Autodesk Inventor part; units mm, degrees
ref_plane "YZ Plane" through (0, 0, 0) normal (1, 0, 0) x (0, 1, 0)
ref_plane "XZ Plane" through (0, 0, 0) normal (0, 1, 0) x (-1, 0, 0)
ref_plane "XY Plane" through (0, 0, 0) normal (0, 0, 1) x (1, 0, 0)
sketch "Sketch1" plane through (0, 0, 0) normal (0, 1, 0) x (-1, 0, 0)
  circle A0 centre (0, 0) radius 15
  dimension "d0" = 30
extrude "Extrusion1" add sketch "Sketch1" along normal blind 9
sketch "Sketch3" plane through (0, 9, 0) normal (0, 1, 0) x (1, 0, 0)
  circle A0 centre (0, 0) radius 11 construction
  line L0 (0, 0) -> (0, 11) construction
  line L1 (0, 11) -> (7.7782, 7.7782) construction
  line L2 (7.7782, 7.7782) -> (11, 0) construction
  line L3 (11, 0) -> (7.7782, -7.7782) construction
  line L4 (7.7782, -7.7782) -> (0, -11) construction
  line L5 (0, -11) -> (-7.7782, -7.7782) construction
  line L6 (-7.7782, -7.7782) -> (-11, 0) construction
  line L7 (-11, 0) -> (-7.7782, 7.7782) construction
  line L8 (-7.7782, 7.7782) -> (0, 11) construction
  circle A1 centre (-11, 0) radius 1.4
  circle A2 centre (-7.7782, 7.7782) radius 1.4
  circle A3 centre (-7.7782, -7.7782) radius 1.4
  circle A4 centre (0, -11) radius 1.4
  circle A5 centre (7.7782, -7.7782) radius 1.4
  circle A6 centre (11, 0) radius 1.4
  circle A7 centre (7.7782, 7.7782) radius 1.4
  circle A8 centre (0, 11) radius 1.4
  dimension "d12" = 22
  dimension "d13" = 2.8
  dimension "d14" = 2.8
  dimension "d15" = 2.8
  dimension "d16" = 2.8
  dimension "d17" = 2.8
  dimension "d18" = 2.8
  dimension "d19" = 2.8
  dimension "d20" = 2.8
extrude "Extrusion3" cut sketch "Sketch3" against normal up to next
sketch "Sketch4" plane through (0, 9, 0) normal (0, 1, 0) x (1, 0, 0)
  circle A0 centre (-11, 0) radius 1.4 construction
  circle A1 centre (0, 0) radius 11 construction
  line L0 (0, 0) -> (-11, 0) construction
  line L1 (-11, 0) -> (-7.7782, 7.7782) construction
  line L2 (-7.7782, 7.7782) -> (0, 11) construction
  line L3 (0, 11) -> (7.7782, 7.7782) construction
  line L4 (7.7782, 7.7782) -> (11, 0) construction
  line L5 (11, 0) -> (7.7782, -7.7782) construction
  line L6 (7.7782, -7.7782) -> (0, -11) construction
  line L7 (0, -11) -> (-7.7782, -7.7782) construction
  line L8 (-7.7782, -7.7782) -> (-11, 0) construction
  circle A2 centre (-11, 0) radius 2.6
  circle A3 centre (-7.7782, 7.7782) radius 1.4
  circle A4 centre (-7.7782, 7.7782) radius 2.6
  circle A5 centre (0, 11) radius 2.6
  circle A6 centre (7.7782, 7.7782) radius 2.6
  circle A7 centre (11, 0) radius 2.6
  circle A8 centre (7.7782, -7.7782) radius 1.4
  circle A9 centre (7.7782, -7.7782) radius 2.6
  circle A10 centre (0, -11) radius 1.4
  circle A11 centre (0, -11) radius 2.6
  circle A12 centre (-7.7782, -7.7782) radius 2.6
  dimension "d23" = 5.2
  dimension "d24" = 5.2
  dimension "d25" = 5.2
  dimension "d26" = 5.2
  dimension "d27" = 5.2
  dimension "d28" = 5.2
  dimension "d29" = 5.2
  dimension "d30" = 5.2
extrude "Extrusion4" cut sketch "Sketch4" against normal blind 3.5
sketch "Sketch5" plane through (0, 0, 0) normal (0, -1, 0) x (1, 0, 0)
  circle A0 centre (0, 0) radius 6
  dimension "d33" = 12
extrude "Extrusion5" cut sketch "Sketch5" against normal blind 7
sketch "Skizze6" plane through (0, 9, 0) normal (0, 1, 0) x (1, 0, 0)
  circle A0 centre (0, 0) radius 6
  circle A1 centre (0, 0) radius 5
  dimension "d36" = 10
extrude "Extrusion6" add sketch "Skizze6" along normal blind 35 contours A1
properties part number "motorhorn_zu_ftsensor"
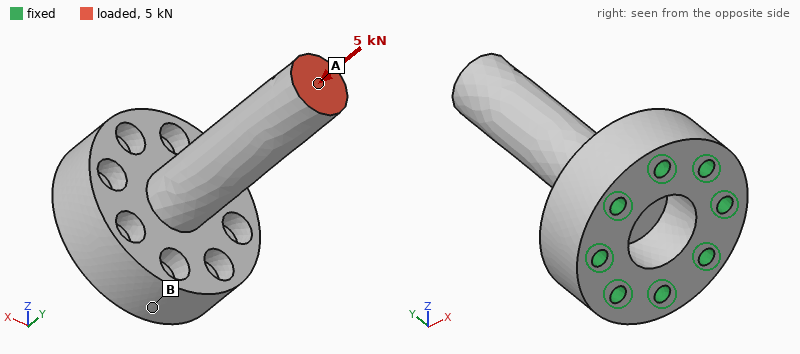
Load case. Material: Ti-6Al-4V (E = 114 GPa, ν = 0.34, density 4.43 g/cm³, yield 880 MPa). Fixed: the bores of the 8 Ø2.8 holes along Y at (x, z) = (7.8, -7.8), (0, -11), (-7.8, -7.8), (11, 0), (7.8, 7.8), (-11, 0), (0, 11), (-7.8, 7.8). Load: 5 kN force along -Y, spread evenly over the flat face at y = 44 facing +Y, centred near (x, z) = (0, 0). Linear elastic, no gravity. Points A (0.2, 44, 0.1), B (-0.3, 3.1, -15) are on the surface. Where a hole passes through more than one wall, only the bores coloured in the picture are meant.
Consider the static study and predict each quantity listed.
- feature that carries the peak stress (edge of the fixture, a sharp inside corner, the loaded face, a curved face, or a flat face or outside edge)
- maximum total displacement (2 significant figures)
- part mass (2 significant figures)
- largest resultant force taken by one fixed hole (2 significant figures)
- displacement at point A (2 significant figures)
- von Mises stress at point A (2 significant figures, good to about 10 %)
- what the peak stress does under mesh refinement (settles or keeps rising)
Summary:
a sharp inside corner
28 µm
33 g
840 N
28 µm
64 MPa
keeps rising
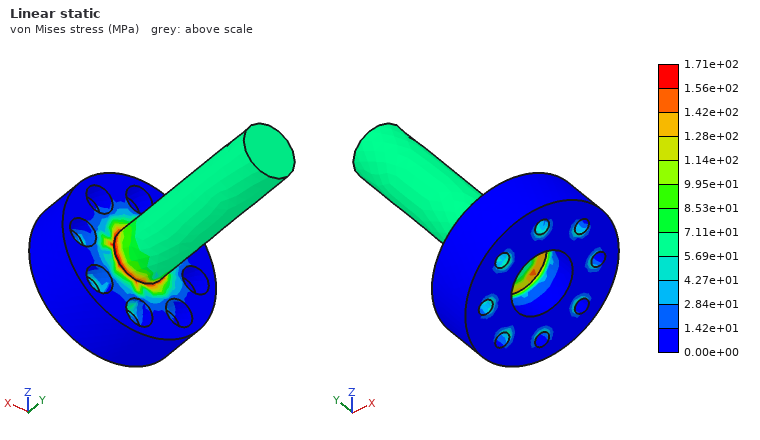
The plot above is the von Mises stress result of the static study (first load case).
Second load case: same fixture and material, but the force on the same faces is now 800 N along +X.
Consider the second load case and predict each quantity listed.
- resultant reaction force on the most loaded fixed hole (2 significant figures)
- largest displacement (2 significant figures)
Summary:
1.0 kN
0.31 mm
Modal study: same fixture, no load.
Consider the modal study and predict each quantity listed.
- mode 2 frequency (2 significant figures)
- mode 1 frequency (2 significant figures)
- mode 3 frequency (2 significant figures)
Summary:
4400 Hz
4400 Hz
21 kHz
